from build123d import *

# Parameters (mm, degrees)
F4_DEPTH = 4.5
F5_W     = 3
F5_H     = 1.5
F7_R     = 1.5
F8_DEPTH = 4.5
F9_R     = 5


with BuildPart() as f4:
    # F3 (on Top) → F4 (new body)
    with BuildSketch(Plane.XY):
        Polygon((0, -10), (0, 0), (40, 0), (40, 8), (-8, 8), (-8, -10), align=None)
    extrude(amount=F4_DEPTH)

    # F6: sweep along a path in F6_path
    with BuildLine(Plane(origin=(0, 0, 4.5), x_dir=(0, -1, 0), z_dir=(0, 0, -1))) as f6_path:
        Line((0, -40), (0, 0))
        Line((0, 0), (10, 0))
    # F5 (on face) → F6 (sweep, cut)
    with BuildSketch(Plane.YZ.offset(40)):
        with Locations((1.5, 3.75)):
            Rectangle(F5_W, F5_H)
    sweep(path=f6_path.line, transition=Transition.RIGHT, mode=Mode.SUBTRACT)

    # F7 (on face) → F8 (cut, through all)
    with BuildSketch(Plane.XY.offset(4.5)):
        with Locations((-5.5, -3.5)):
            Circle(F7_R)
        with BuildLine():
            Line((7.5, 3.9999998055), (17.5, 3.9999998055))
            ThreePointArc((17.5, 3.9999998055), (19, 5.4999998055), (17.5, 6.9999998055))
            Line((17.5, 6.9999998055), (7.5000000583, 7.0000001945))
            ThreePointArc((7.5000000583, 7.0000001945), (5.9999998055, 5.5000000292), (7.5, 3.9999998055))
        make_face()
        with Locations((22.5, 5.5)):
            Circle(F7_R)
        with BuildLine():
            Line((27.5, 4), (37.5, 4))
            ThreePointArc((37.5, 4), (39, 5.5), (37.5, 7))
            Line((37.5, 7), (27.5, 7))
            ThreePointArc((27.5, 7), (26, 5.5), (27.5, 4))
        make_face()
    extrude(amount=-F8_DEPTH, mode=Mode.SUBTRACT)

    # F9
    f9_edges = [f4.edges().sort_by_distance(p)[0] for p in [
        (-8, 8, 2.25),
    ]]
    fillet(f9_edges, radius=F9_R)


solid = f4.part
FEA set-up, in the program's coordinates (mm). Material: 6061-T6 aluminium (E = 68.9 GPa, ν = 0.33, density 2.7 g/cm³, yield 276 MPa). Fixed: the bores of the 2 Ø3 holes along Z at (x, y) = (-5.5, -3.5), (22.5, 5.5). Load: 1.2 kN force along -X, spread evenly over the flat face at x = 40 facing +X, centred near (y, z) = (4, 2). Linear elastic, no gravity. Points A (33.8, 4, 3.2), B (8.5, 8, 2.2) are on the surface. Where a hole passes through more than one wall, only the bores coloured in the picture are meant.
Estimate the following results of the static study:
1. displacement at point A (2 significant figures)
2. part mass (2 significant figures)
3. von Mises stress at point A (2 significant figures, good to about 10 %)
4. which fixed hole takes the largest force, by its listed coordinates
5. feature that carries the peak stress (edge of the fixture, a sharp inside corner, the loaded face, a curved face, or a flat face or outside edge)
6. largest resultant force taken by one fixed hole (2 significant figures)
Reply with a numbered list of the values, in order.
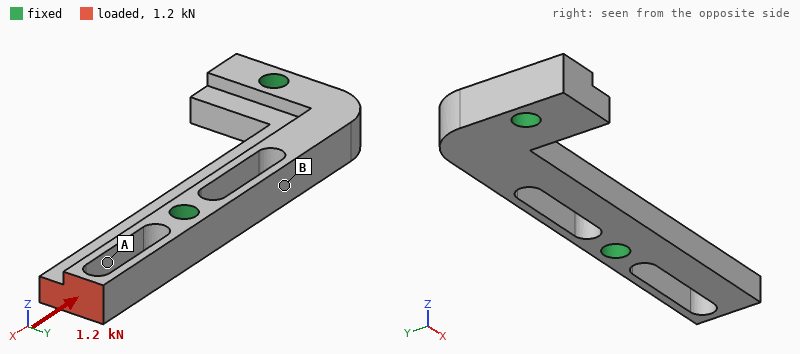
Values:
1. 14 µm
2. 3.9 g
3. 110 MPa
4. (22.5, 5.5)
5. a curved face
6. 1.2 kN
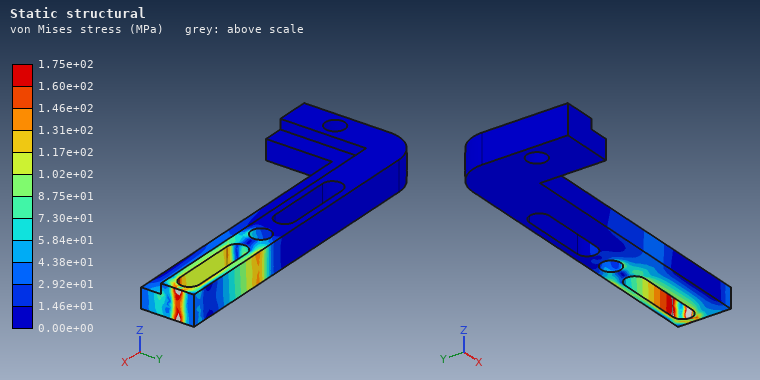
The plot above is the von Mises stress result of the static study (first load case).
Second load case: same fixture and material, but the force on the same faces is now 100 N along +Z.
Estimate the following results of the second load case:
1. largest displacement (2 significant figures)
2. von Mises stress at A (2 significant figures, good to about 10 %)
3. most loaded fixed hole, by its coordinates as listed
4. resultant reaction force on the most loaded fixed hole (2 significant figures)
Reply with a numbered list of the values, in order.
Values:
1. 91 µm
2. 36 MPa
3. (22.5, 5.5)
4. 100 N
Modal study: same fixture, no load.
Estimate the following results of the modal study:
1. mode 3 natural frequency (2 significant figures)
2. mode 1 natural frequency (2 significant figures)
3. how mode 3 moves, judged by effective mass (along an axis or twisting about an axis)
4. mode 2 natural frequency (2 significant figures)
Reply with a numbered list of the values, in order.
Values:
1. 19 kHz
2. 10 kHz
3. along Z
4. 12 kHz
